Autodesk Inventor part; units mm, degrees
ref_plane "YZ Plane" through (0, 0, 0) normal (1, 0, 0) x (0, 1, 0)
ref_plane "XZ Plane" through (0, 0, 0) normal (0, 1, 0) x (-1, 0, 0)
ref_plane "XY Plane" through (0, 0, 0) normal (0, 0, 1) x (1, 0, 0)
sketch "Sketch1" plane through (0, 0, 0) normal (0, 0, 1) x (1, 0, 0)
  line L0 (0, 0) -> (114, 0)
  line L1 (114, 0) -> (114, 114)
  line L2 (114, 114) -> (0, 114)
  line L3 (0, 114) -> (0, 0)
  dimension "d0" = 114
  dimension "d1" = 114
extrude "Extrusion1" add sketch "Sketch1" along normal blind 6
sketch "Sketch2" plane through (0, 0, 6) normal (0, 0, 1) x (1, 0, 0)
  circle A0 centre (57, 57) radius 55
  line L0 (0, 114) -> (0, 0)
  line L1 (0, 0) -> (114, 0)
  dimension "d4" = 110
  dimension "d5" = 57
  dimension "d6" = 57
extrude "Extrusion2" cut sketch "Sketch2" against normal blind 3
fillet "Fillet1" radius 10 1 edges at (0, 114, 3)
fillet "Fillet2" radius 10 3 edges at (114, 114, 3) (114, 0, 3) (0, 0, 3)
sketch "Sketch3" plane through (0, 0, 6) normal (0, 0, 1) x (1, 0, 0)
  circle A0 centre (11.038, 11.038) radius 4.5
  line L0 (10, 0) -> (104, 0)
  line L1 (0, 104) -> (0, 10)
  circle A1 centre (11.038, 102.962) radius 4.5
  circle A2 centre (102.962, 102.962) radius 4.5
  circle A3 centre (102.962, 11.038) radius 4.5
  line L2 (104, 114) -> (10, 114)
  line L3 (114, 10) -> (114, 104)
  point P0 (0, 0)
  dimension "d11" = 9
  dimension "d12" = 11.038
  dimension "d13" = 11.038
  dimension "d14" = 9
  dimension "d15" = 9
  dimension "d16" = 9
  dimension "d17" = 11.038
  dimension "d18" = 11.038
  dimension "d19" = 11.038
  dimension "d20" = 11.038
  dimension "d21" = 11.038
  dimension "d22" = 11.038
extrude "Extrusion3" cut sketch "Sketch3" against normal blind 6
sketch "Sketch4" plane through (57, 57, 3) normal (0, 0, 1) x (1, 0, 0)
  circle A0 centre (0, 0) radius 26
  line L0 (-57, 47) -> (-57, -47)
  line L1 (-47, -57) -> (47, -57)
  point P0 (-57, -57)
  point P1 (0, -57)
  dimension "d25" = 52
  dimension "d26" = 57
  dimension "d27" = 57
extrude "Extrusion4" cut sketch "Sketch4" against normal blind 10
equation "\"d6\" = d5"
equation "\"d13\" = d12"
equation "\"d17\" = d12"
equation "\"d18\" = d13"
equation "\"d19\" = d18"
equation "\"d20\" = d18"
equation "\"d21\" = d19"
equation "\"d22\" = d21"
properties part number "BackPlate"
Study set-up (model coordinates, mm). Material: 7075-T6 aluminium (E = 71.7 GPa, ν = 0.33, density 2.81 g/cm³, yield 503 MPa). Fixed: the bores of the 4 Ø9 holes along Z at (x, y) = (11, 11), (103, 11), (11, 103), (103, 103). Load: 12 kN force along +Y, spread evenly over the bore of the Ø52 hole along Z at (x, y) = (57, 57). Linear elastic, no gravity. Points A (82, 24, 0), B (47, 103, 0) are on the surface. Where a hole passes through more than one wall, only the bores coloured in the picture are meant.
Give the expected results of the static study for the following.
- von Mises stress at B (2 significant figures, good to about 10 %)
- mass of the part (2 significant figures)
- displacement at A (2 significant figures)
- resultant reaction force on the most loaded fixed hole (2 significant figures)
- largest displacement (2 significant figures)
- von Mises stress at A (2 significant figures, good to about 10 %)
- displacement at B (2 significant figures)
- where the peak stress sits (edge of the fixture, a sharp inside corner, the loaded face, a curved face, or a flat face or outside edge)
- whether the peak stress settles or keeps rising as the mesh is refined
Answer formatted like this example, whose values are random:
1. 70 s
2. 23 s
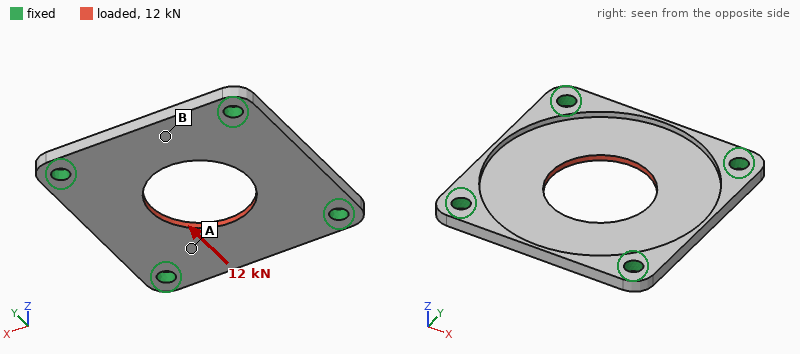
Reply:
1. 17 MPa
2. 120 g
3. 21 µm
4. 3.2 kN
5. 38 µm
6. 30 MPa
7. 30 µm
8. edge of the fixture
9. keeps rising
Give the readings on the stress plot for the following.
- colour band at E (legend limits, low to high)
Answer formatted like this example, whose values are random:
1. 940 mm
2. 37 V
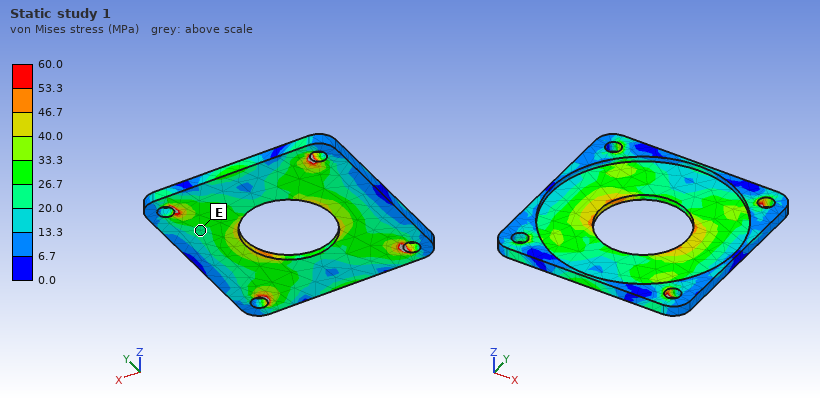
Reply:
1. 20.0 to 26.7 MPa
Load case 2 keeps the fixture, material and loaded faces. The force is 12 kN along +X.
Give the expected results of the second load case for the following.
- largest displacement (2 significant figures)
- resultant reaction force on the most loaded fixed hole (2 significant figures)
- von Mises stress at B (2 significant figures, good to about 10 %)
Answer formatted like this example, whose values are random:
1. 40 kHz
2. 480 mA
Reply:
1. 39 µm
2. 3.2 kN
3. 18 MPa
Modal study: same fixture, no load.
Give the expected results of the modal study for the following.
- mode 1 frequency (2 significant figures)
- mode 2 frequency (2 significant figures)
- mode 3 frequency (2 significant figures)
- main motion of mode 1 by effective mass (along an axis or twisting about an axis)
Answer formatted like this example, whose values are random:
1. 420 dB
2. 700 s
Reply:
1. 2600 Hz
2. 3400 Hz
3. 3400 Hz
4. along Z
